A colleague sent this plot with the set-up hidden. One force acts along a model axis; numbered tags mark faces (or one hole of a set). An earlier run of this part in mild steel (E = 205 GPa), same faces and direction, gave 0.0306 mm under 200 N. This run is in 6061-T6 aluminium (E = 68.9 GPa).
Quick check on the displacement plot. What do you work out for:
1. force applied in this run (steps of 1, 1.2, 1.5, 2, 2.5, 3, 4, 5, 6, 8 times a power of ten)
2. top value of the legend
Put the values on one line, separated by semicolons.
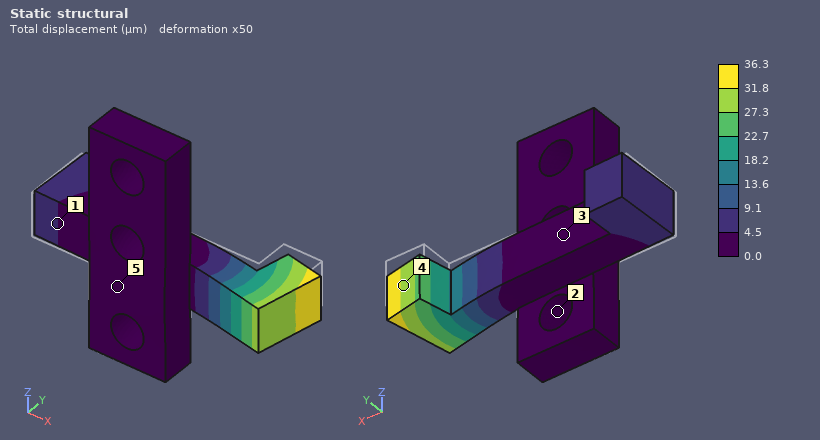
80 N; 36.3 µm
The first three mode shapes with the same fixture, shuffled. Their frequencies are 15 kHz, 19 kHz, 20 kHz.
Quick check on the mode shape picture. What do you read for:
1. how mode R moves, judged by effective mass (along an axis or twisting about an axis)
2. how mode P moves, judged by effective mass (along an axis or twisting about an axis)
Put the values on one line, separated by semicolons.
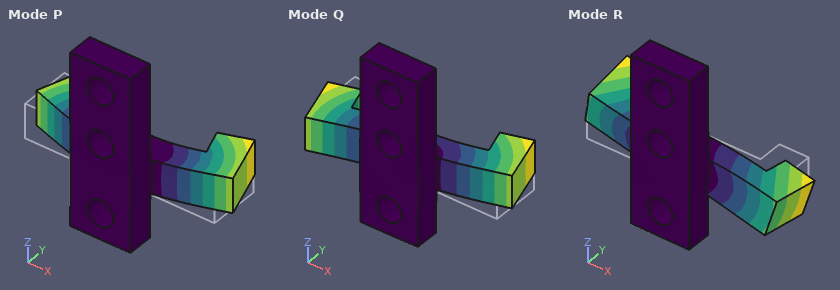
twisting about Y; along Y
